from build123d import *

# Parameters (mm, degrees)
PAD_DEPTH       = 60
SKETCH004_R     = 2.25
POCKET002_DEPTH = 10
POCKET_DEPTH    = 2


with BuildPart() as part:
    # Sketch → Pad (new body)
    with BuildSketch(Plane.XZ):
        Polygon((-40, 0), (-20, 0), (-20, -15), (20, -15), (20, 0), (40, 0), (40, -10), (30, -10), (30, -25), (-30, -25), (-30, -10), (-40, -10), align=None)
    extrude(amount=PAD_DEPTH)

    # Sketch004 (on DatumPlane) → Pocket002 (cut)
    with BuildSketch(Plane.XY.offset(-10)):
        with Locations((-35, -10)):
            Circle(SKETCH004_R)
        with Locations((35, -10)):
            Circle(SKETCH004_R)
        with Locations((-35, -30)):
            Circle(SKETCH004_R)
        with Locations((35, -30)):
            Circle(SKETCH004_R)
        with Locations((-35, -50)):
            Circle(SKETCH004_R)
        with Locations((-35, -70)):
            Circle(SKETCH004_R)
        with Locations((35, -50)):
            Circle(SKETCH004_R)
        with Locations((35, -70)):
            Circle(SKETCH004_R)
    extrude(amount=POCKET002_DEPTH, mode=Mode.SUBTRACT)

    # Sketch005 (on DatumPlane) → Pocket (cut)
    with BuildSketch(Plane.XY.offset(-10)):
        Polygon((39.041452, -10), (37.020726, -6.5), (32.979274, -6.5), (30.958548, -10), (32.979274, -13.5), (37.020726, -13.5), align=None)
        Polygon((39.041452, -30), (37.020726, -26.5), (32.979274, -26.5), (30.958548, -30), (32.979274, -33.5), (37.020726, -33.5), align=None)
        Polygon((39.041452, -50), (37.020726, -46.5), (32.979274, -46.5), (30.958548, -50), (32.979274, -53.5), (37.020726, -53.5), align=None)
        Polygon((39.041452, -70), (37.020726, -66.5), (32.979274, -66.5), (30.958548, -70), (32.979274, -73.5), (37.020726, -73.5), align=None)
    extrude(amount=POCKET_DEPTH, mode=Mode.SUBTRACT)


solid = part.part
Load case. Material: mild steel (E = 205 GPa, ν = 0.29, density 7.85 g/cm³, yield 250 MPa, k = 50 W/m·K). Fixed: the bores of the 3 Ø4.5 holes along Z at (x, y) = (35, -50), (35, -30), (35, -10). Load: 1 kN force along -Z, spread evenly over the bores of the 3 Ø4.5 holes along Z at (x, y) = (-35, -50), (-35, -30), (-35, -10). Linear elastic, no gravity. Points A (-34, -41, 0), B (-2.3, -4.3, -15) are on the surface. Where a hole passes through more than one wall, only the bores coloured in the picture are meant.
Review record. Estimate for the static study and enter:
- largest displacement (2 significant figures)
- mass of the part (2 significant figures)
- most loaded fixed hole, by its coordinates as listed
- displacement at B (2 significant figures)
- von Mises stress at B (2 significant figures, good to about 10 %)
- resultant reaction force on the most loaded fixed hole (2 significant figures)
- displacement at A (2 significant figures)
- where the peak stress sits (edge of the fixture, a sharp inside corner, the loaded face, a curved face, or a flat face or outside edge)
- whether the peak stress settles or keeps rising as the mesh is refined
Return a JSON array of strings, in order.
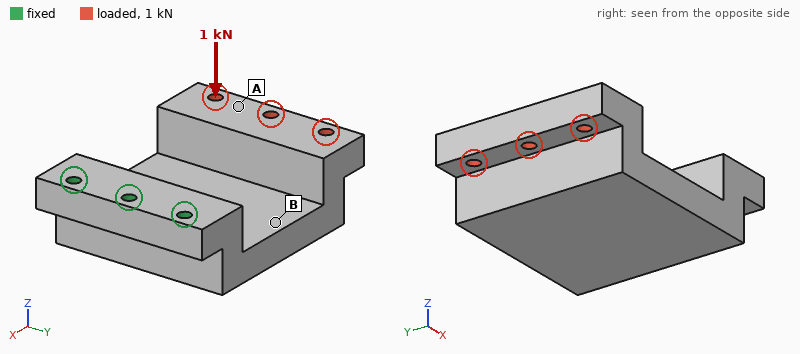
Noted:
["0.18 mm", "510 g", "(35, -30)", "0.063 mm", "32 MPa", "510 N", "0.16 mm", "edge of the fixture", "keeps rising"]
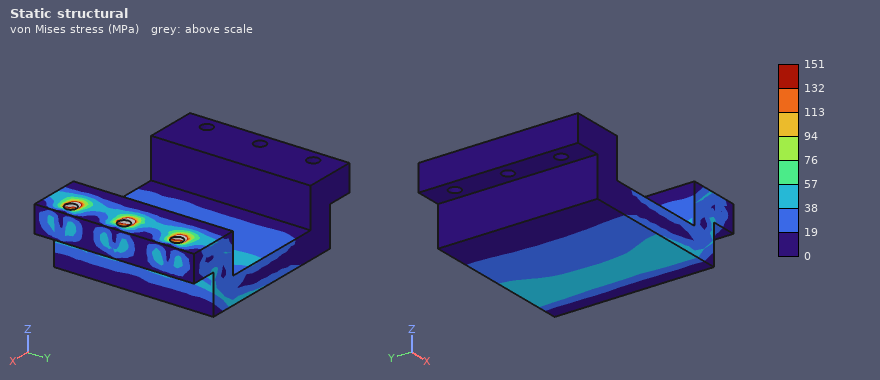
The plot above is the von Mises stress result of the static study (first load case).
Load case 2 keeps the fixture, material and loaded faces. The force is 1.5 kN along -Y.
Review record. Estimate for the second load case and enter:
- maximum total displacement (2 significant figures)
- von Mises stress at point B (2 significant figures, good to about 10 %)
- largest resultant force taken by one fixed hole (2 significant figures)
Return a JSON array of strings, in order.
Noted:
["56 µm", "23 MPa", "2.4 kN"]
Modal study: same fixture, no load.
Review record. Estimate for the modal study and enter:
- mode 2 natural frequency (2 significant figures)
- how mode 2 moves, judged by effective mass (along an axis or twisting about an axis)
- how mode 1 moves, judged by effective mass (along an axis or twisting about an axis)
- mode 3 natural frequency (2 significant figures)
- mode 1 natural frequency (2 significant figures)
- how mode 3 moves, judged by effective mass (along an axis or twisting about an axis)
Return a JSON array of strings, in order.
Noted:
["2300 Hz", "along Y", "along Z", "4100 Hz", "980 Hz", "along X"]
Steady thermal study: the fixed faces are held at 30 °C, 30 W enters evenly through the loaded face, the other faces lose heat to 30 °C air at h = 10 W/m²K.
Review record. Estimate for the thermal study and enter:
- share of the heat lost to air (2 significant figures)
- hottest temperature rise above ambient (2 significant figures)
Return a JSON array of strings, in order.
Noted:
["20 %", "77 K"]
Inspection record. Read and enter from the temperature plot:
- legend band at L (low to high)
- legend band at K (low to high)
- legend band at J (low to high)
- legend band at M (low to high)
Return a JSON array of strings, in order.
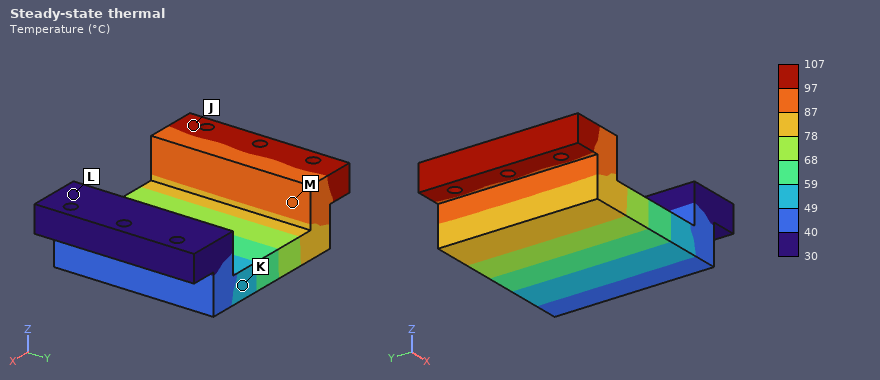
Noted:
["30 to 40 °C", "49 to 59 °C", "97 to 107 °C", "87 to 97 °C"]
